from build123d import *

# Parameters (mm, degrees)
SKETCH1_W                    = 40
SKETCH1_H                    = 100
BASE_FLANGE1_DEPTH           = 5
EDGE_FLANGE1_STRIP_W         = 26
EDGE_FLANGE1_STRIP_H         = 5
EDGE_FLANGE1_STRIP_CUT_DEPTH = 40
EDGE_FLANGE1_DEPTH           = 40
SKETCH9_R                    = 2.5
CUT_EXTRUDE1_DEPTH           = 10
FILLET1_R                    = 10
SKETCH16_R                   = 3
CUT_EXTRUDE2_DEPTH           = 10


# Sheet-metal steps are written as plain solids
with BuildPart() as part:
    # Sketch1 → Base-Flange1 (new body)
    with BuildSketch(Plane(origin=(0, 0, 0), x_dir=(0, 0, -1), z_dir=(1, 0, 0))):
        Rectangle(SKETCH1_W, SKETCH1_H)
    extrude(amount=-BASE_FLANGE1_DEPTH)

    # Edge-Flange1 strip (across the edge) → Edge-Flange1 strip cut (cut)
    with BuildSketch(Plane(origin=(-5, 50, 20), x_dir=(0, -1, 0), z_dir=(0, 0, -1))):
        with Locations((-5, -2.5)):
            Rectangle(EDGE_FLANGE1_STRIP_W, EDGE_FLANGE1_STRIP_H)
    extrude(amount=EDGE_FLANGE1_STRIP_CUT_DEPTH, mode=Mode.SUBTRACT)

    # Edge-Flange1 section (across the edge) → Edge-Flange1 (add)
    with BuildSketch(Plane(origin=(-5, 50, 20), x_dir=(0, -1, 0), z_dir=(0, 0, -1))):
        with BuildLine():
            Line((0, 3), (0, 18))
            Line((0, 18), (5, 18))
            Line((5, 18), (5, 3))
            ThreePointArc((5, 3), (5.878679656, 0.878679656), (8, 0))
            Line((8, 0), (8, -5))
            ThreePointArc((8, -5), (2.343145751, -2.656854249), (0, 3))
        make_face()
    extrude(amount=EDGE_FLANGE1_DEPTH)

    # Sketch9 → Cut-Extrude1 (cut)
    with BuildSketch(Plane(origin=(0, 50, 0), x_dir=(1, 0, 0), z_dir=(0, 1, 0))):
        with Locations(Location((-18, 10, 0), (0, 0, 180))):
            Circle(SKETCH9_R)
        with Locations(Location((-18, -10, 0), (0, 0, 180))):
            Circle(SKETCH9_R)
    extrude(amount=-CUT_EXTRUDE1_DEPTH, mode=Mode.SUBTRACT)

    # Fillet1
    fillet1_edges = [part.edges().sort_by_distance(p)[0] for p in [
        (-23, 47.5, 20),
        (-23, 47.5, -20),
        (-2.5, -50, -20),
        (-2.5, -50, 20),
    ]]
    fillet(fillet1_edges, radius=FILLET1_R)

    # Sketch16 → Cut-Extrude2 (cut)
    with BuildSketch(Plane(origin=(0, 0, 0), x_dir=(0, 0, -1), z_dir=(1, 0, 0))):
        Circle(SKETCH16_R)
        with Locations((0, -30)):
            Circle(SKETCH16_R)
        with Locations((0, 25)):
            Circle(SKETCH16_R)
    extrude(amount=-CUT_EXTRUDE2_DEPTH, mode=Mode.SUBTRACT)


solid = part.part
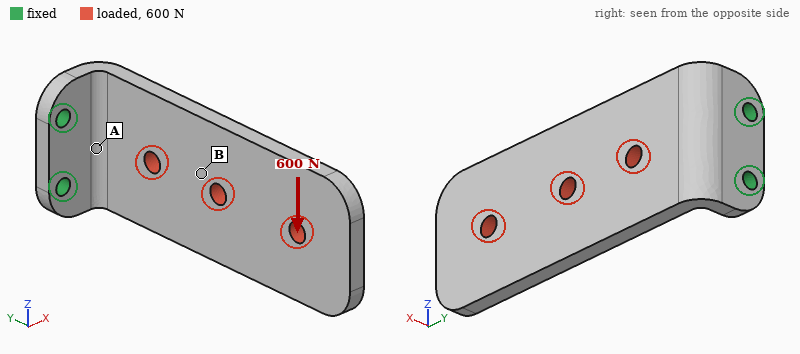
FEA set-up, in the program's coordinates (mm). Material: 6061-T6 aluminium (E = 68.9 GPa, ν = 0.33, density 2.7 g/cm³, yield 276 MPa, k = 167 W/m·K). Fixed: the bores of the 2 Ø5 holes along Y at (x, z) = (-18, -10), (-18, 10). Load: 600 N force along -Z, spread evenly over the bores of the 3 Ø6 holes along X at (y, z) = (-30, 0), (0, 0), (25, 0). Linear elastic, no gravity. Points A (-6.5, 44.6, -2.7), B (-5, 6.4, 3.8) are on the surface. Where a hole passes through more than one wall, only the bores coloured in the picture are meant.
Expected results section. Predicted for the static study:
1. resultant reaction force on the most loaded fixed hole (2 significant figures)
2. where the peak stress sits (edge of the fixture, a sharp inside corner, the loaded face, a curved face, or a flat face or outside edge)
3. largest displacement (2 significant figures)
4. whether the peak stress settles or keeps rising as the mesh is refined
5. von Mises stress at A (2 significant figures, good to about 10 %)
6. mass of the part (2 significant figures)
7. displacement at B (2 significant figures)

1.3 kN
edge of the fixture
0.42 mm
keeps rising
92 MPa
60 g
0.18 mm
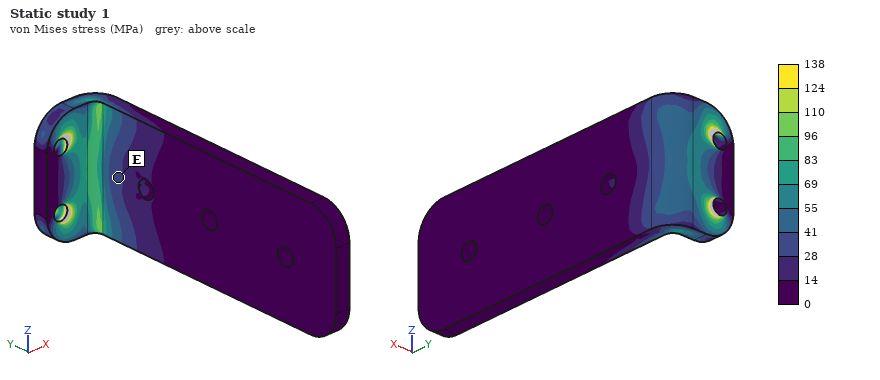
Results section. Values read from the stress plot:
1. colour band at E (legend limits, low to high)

28 to 41 MPa
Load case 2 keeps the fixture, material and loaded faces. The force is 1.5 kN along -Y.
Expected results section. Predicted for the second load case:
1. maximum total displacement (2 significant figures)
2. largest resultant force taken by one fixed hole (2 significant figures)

0.60 mm
750 N
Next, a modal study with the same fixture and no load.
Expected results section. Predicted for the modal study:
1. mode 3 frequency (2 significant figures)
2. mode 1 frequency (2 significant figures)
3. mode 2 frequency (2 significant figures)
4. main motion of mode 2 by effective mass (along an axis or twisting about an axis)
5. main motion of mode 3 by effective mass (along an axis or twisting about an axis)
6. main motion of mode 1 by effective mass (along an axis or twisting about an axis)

2100 Hz
360 Hz
1000 Hz
along Z
twisting about Y
along X
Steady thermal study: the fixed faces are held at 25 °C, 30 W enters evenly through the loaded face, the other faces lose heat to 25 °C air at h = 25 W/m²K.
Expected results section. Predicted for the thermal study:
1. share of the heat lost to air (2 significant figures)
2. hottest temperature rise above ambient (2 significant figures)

24 %
45 K
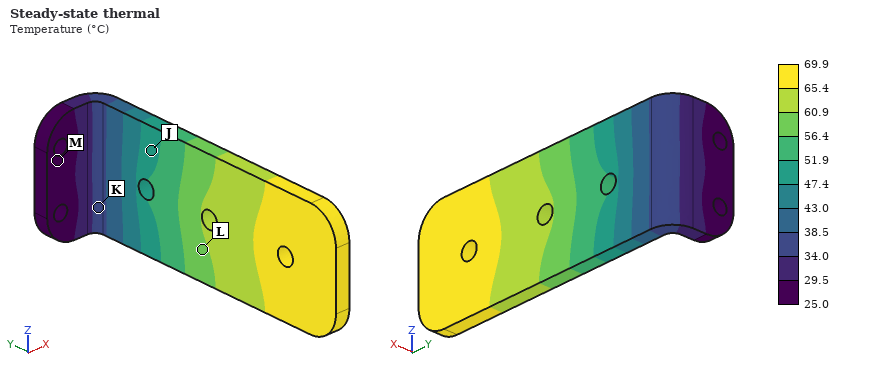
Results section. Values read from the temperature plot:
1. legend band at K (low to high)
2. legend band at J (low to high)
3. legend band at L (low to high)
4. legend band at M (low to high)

34.0 to 38.5 °C
47.4 to 51.9 °C
56.4 to 60.9 °C
25.0 to 29.5 °C
